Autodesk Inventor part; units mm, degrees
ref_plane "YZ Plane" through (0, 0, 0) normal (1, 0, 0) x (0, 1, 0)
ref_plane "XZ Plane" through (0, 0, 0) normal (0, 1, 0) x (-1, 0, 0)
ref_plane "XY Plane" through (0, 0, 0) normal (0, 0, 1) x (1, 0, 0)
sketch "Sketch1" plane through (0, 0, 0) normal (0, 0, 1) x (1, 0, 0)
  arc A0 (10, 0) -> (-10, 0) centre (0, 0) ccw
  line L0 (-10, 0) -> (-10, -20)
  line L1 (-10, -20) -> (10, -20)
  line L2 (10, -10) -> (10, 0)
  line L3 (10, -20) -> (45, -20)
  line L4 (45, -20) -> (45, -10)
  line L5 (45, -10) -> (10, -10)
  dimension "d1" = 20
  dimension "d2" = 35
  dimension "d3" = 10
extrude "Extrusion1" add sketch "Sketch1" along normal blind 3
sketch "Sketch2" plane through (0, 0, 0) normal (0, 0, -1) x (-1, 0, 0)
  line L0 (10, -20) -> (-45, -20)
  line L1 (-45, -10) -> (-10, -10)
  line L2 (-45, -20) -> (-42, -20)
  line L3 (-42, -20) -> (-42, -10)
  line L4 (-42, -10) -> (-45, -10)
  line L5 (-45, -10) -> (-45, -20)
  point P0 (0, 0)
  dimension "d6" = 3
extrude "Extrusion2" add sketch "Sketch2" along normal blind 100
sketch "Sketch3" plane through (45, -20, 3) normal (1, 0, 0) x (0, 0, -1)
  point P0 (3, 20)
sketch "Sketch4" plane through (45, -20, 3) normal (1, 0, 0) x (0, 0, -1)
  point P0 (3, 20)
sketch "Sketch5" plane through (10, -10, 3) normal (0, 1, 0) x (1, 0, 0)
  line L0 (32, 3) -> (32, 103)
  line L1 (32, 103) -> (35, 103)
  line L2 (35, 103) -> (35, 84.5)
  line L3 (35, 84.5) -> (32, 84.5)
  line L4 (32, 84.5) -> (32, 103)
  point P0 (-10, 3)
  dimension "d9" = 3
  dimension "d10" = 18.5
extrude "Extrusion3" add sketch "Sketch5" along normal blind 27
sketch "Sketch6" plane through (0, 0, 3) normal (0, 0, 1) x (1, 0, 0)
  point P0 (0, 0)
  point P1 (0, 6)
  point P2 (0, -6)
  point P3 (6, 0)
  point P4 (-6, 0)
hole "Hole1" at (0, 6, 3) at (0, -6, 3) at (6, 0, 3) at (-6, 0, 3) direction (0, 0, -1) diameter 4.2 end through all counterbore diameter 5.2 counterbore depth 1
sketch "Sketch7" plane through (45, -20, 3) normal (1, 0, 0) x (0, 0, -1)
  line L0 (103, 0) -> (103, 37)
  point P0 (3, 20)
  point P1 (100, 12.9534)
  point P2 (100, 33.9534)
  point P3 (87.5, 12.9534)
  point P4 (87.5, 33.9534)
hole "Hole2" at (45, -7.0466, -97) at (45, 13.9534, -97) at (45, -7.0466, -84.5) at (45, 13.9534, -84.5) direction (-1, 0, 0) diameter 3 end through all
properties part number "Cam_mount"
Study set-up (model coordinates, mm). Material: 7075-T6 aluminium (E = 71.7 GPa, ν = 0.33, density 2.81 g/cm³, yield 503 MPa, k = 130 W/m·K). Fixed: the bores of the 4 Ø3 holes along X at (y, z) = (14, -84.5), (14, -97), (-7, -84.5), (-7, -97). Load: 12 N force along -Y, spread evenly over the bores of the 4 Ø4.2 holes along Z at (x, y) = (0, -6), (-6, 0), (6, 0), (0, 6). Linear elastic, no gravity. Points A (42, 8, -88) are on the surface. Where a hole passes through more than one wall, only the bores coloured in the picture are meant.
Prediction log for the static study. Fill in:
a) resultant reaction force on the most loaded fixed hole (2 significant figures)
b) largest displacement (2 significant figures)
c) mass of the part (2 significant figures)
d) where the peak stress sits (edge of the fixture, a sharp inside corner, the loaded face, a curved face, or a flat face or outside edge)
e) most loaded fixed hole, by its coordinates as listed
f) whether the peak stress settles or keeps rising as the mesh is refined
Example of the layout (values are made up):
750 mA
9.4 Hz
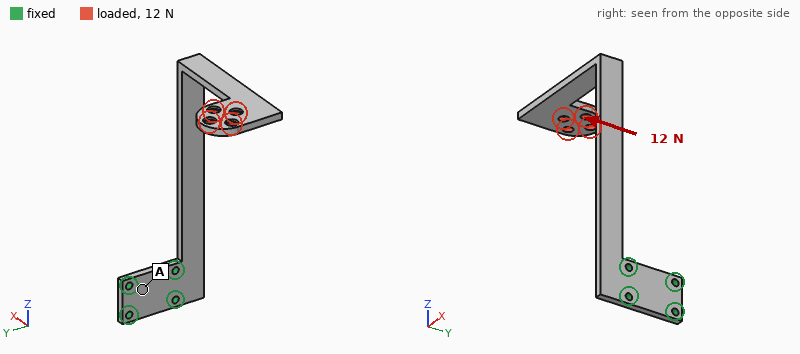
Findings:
97 N
1.4 mm
19 g
a sharp inside corner
(-7, -84.5)
keeps rising
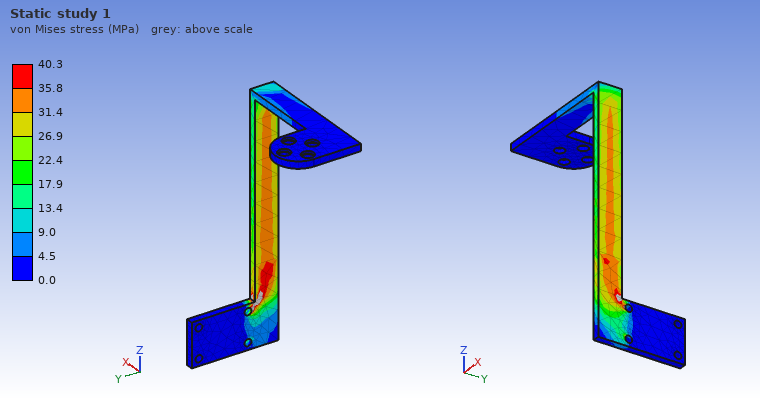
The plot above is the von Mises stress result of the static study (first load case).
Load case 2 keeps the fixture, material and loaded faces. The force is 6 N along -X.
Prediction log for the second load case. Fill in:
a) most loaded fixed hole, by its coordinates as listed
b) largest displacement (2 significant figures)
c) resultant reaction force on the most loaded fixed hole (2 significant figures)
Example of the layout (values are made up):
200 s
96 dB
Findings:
(-7, -84.5)
1.2 mm
31 N
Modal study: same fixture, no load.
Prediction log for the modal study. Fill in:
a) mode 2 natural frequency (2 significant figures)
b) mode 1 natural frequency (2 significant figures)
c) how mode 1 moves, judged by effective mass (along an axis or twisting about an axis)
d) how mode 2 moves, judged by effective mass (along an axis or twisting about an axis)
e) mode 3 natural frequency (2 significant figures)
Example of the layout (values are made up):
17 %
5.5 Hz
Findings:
230 Hz
120 Hz
along X
along Y
400 Hz
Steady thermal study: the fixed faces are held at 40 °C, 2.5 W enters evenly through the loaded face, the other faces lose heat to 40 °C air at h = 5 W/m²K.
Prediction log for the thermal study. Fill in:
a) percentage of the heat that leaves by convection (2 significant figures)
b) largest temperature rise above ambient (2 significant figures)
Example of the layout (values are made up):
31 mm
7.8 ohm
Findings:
34 %
64 K
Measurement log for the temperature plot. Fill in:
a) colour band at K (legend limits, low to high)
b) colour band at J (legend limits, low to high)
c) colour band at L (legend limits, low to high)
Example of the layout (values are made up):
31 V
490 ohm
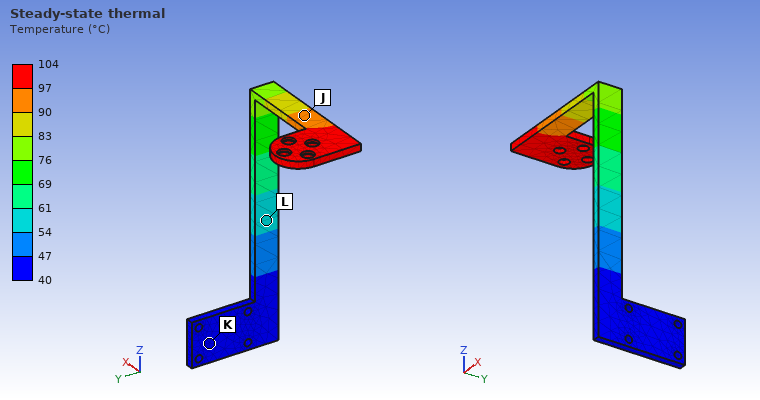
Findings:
40 to 47 °C
90 to 97 °C
54 to 61 °C
